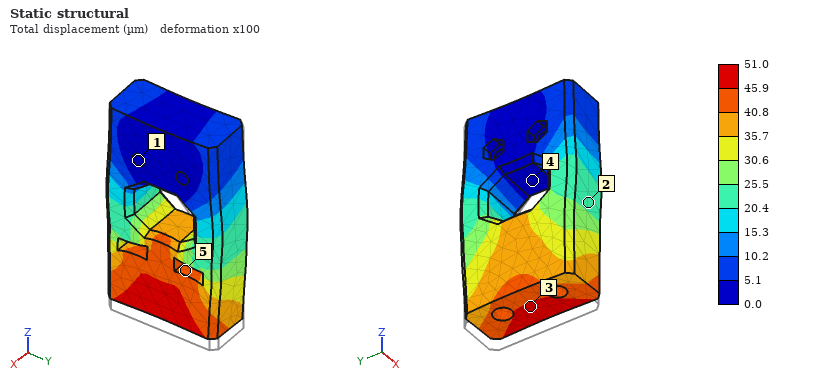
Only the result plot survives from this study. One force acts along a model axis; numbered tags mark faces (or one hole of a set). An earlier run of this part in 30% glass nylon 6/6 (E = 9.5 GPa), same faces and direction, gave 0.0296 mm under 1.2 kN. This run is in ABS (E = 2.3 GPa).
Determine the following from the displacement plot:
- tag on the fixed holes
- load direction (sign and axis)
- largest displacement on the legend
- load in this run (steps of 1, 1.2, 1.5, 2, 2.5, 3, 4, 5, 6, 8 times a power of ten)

1
+Z
51.0 µm
500 N
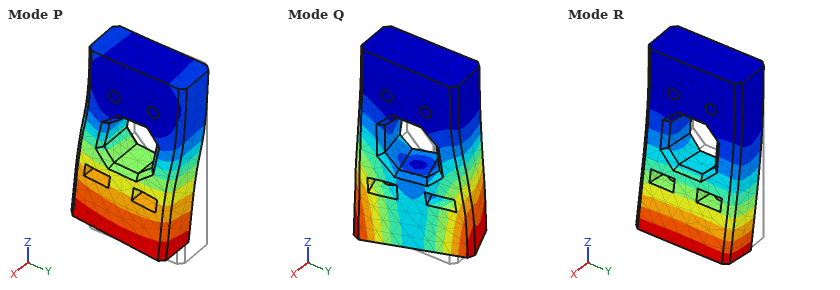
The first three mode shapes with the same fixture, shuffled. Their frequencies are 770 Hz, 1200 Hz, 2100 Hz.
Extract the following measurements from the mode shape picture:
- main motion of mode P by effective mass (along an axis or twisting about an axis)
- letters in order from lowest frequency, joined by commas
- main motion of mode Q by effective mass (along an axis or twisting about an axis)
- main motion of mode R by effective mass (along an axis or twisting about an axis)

along Y
R, P, Q
twisting about Z
along X
